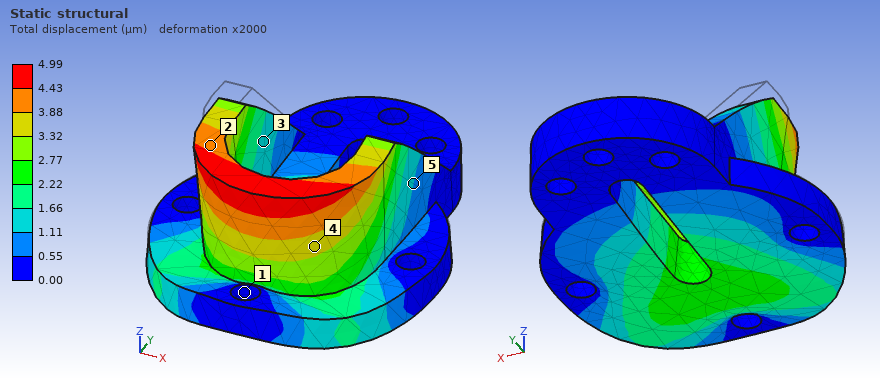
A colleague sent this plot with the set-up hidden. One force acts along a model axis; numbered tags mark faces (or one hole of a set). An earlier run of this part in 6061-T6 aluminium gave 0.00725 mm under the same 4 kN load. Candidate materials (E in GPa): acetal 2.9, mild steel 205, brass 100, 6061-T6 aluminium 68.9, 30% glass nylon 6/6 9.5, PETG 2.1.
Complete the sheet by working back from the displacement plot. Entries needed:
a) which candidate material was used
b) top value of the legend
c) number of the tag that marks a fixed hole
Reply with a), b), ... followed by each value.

a) brass
b) 4.99 µm
c) 1
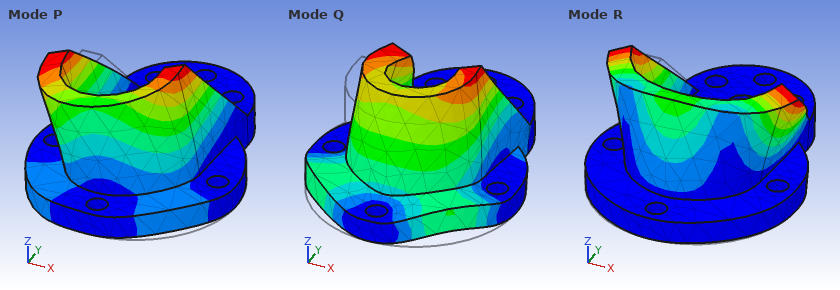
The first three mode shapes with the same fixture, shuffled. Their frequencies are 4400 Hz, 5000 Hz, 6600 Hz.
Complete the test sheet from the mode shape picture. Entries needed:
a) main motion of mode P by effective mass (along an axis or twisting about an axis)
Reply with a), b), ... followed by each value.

a) along X
